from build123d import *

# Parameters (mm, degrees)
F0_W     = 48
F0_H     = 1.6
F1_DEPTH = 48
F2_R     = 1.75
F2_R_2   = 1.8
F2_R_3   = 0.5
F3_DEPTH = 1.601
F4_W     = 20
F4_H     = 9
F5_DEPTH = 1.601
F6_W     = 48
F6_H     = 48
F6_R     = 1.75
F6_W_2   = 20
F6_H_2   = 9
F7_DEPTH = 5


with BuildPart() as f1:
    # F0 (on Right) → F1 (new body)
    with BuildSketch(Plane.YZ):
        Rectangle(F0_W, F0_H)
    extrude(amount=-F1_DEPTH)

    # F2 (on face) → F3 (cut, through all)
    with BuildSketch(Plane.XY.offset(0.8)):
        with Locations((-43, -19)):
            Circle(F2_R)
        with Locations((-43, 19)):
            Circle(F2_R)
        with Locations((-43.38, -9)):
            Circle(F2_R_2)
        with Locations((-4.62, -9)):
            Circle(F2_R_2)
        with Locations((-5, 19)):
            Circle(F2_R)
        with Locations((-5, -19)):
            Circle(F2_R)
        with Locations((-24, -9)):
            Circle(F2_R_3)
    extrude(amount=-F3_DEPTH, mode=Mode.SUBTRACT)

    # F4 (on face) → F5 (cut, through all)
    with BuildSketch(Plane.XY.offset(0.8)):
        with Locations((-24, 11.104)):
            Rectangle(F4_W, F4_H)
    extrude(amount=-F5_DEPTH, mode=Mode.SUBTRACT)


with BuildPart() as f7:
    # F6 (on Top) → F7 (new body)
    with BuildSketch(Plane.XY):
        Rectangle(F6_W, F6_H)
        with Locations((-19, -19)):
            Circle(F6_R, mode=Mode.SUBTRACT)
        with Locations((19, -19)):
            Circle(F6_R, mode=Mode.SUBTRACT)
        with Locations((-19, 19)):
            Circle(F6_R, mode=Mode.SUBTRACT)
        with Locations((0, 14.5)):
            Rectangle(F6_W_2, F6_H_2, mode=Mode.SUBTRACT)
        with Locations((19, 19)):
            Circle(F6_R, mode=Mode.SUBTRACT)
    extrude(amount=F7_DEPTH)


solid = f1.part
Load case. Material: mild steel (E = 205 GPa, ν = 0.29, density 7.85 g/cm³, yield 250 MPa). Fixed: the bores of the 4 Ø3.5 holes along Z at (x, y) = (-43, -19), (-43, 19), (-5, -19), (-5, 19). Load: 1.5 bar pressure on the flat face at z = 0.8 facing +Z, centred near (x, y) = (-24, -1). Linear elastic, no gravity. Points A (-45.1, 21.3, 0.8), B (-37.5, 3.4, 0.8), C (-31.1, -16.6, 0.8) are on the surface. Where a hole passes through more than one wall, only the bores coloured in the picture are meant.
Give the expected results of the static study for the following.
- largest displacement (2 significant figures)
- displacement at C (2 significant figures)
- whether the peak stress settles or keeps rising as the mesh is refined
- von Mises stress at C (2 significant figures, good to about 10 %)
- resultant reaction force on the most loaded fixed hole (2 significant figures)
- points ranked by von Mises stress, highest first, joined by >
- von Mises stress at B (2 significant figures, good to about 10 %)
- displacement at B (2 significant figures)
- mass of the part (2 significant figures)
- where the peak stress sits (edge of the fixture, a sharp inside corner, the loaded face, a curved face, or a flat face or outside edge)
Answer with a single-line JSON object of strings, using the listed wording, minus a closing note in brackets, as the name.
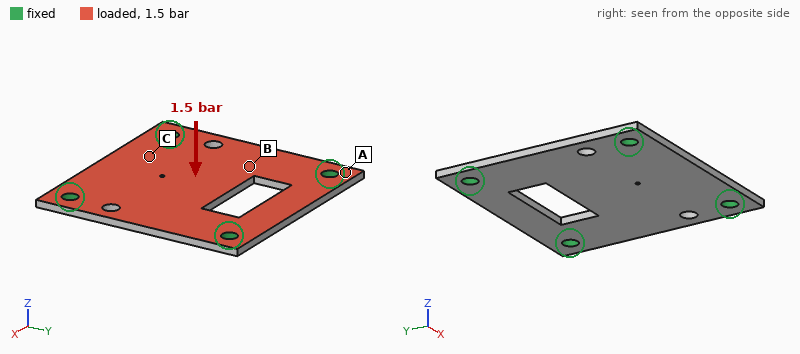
{"largest displacement": "28 µm", "displacement at C": "11 µm", "whether the peak stress settles or keeps rising as the mesh is refined": "keeps rising", "von Mises stress at C": "16 MPa", "resultant reaction force on the most loaded fixed hole": "81 N", "points ranked by von Mises stress, highest first, joined by >": "B > C > A", "von Mises stress at B": "24 MPa", "displacement at B": "17 µm", "mass of the part": "26 g", "where the peak stress sits": "edge of the fixture"}
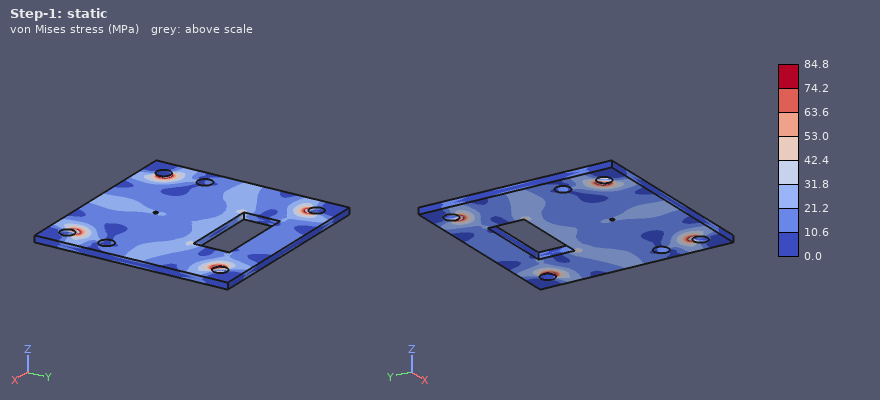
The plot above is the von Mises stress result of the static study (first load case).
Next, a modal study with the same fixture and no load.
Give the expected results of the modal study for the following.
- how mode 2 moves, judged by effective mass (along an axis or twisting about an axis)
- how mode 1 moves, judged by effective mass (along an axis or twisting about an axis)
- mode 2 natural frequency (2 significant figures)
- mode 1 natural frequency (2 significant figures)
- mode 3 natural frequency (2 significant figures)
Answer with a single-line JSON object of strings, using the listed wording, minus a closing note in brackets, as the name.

{"how mode 2 moves, judged by effective mass": "twisting about Y", "how mode 1 moves, judged by effective mass": "along Z", "mode 2 natural frequency": "6800 Hz", "mode 1 natural frequency": "4200 Hz", "mode 3 natural frequency": "7100 Hz"}
